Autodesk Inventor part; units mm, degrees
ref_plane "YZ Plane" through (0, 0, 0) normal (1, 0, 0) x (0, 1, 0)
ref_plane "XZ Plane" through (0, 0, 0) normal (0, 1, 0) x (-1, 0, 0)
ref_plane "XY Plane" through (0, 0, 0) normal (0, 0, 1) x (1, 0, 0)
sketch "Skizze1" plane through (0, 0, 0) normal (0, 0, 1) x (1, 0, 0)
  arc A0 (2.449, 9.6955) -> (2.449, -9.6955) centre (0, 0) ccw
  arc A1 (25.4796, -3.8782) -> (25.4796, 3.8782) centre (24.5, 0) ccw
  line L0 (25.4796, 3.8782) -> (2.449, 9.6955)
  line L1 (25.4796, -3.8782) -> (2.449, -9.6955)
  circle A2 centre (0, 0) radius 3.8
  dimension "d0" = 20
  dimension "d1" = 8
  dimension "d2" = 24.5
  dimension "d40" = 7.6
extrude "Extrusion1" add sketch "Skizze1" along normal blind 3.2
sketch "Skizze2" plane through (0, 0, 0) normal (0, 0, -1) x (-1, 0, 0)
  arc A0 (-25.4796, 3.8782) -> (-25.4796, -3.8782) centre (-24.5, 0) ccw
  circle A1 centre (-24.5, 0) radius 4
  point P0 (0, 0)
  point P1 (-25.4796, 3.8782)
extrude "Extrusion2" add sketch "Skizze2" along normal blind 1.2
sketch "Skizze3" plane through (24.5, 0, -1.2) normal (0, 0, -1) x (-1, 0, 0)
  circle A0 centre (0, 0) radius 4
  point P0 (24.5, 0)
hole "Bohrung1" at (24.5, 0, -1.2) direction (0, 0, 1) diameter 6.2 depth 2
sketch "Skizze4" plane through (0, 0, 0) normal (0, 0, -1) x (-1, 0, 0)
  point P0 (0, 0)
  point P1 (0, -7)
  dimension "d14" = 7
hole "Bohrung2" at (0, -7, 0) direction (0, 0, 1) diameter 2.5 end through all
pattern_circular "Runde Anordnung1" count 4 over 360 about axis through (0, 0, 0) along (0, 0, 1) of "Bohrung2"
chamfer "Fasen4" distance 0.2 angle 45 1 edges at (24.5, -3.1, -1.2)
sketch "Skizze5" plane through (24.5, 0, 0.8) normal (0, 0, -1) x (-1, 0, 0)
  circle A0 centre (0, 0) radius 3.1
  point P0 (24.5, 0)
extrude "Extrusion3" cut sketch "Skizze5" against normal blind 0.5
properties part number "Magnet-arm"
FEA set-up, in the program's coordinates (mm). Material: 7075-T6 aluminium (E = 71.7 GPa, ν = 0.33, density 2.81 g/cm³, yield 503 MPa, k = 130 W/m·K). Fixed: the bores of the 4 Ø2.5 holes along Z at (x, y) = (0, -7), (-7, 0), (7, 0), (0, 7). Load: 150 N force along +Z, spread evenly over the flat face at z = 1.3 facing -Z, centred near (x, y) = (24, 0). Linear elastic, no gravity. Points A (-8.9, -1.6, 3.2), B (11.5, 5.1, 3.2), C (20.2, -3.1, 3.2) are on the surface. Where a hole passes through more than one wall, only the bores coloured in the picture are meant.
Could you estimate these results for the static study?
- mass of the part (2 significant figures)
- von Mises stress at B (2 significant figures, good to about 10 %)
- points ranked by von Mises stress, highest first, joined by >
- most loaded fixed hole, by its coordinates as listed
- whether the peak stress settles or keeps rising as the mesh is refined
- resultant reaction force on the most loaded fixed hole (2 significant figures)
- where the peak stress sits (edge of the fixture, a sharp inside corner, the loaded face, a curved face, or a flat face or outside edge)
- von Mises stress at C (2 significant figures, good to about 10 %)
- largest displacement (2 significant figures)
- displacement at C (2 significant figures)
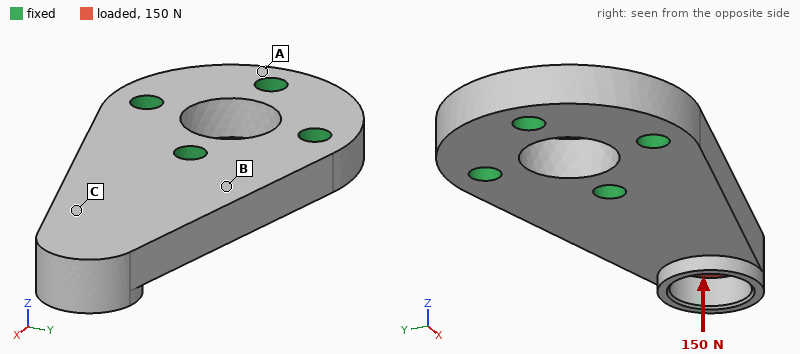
4.2 g
70 MPa
B > C > A
(7, 0)
keeps rising
290 N
edge of the fixture
41 MPa
0.14 mm
0.064 mm
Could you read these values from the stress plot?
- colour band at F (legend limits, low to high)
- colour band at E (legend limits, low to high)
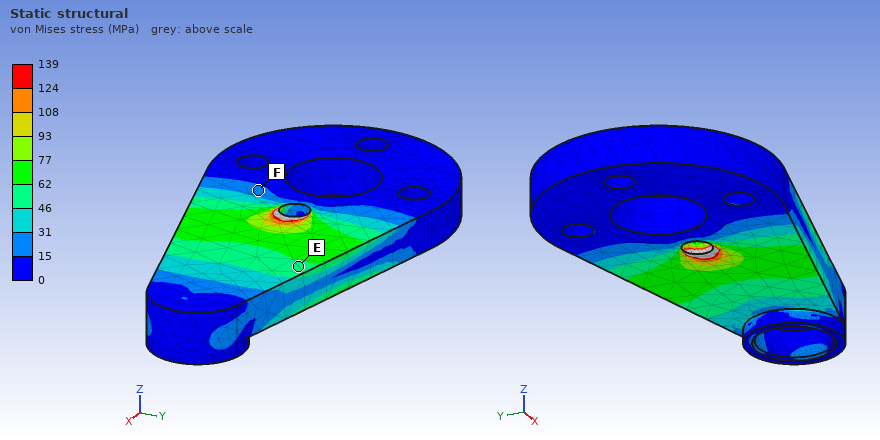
15 to 31 MPa
46 to 62 MPa
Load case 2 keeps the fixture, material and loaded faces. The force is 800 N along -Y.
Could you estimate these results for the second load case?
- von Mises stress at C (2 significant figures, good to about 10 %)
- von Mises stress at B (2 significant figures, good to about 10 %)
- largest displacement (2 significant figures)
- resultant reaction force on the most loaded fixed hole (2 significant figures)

52 MPa
67 MPa
79 µm
870 N
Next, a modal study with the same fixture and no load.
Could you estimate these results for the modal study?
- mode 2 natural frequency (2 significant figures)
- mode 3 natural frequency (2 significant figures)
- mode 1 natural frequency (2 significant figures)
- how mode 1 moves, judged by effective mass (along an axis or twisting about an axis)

23 kHz
24 kHz
7700 Hz
along Z
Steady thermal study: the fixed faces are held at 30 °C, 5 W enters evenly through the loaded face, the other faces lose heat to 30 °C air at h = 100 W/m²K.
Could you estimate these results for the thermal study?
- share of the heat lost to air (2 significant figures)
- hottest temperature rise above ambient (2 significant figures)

12 %
19 K
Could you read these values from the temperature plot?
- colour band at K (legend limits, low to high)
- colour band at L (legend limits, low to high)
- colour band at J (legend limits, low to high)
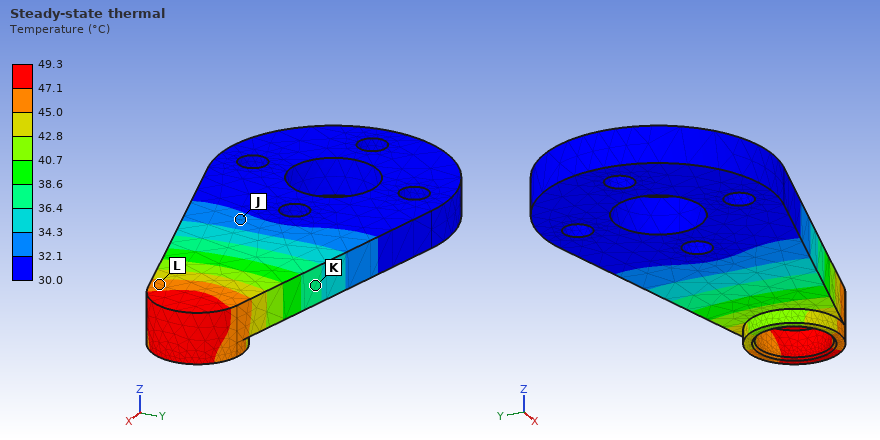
36.4 to 38.6 °C
45.0 to 47.1 °C
32.1 to 34.3 °C
